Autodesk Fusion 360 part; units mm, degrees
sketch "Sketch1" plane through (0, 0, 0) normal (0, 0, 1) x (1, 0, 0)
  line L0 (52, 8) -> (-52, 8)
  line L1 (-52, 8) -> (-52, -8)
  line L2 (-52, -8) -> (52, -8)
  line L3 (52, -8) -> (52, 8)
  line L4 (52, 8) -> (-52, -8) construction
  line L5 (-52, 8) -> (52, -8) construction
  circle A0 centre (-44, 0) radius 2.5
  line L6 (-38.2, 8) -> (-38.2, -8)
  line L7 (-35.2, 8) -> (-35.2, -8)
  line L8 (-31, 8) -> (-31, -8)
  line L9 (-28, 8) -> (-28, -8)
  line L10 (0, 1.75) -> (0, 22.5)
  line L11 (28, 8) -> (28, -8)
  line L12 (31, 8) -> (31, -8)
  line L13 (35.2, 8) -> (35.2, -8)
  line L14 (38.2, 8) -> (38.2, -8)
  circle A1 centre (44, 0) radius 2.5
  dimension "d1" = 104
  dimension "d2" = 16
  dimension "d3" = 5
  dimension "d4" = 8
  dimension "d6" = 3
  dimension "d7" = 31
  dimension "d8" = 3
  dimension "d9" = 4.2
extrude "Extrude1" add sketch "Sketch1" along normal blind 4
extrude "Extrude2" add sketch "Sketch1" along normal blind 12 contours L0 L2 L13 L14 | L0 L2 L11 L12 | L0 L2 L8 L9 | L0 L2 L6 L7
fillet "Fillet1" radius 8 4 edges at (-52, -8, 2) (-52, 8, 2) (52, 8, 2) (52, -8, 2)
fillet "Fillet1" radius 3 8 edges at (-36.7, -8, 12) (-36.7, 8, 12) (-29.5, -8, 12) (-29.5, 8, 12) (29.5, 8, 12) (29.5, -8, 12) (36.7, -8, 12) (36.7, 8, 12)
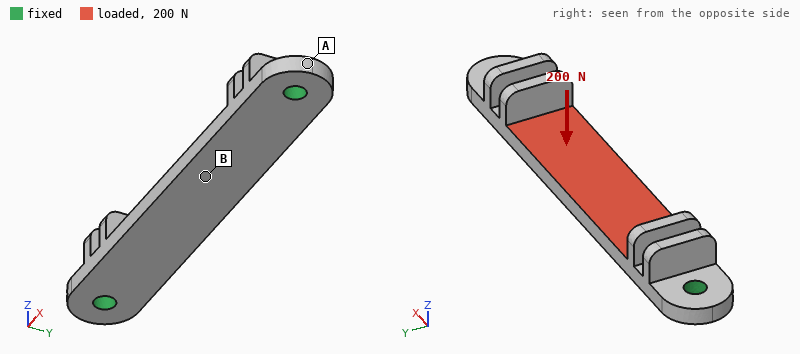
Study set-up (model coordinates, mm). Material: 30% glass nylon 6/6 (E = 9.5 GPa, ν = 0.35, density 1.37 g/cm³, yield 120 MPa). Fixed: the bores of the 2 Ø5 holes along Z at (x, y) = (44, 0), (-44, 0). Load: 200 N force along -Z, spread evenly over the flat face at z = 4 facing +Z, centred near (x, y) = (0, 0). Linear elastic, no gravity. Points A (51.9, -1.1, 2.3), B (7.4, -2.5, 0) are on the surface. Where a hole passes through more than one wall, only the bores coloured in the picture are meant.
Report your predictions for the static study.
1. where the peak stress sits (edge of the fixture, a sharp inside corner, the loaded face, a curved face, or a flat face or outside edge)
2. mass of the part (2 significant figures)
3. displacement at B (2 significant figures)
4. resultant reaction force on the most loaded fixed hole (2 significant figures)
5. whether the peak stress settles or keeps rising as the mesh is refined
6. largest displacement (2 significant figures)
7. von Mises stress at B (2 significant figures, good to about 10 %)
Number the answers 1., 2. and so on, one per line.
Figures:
1. edge of the fixture
2. 11 g
3. 0.52 mm
4. 100 N
5. keeps rising
6. 0.57 mm
7. 21 MPa
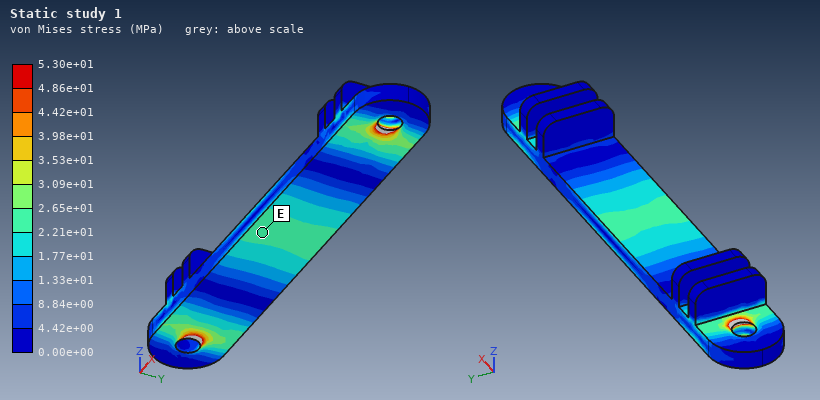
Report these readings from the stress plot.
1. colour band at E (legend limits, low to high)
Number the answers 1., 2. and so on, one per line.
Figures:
1. 2.21e+01 to 2.65e+01 MPa
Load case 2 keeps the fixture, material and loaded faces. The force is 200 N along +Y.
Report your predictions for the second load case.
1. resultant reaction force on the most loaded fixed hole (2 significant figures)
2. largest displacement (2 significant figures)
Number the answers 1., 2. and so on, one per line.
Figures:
1. 100 N
2. 91 µm
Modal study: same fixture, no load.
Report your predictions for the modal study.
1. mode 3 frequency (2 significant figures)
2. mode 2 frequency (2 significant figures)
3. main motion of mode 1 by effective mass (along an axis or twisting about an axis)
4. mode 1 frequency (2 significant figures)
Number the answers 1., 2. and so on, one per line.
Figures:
1. 3800 Hz
2. 3600 Hz
3. along Z
4. 1500 Hz
